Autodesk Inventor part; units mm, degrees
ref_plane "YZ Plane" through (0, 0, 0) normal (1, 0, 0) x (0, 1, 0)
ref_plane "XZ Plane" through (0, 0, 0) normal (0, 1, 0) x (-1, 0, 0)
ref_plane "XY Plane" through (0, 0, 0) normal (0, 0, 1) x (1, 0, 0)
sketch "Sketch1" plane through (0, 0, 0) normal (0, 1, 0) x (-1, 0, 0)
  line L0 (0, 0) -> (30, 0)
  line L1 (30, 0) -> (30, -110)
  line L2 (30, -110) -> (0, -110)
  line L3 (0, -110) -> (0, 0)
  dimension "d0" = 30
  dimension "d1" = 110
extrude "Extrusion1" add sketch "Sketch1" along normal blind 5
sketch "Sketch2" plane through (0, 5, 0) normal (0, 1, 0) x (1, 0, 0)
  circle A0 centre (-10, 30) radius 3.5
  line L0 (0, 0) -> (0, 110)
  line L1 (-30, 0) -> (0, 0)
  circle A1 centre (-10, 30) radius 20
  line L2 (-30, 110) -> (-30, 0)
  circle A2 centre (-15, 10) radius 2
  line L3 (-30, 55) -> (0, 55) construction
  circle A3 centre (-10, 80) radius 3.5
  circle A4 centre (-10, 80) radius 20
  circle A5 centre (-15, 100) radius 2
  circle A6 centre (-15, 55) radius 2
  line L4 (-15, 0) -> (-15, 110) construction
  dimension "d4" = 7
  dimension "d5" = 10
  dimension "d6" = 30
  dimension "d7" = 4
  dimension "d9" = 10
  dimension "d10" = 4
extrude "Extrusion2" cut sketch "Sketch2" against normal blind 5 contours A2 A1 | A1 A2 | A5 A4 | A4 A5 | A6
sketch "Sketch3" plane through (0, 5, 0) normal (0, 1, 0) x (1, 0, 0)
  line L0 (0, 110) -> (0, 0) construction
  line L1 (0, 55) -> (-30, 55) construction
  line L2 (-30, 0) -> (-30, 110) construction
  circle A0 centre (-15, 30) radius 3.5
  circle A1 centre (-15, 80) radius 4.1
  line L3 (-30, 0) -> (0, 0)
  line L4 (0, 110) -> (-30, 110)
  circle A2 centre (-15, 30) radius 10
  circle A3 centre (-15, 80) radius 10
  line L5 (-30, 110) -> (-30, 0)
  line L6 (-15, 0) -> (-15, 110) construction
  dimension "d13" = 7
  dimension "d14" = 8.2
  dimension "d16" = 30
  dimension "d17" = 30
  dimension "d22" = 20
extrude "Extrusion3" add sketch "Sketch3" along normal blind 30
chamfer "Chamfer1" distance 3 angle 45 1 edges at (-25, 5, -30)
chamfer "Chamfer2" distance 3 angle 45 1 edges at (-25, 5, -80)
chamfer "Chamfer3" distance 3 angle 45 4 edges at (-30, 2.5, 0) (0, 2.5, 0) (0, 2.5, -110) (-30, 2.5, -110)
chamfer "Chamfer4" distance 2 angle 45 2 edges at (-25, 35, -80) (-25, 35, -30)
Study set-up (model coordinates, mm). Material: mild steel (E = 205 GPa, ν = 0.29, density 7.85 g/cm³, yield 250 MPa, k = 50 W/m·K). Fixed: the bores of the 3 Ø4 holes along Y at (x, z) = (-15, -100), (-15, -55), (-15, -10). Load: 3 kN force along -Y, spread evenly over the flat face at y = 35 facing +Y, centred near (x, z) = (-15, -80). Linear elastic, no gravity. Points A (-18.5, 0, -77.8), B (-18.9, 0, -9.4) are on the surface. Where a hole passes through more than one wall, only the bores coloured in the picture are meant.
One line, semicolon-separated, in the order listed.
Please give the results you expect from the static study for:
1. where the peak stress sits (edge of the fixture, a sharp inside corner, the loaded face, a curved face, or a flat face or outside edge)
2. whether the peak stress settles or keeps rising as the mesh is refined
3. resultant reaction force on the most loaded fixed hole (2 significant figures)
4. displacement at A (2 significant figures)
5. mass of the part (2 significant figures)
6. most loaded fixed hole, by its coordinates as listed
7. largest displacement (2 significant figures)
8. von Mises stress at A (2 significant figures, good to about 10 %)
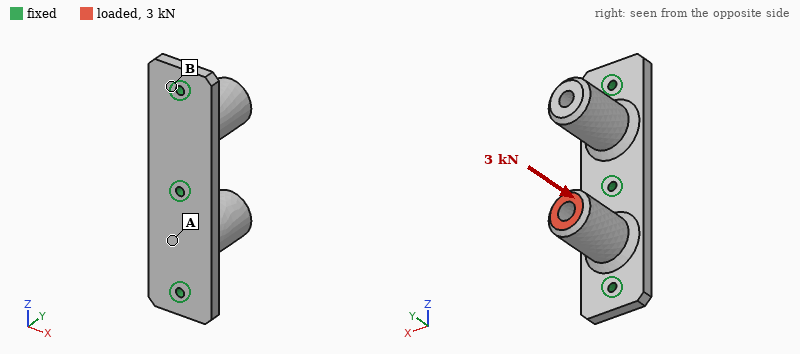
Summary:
edge of the fixture; keeps rising; 1.8 kN; 12 µm; 260 g; (-15, -100); 15 µm; 26 MPa
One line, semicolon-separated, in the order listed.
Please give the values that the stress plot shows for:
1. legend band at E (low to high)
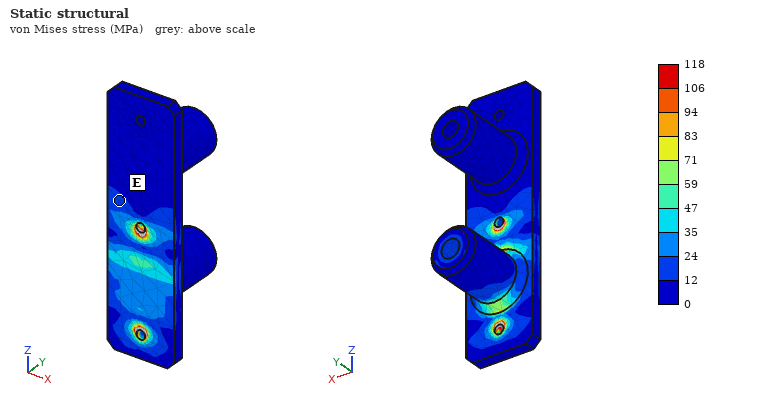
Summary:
12 to 24 MPa
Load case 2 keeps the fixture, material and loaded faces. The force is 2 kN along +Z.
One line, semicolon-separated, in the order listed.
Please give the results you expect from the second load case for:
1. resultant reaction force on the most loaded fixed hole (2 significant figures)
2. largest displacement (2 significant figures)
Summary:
2.1 kN; 43 µm
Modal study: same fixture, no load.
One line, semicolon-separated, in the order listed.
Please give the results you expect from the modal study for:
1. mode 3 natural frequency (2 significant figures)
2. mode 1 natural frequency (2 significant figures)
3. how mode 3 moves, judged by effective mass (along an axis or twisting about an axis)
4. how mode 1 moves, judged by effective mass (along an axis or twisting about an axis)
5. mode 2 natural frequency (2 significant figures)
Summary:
6800 Hz; 3300 Hz; along Z; along X; 3600 Hz
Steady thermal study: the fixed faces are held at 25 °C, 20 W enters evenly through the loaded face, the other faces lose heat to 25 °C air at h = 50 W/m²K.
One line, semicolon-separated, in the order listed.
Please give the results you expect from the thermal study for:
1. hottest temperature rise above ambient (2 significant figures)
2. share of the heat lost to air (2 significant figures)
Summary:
59 K; 35 %
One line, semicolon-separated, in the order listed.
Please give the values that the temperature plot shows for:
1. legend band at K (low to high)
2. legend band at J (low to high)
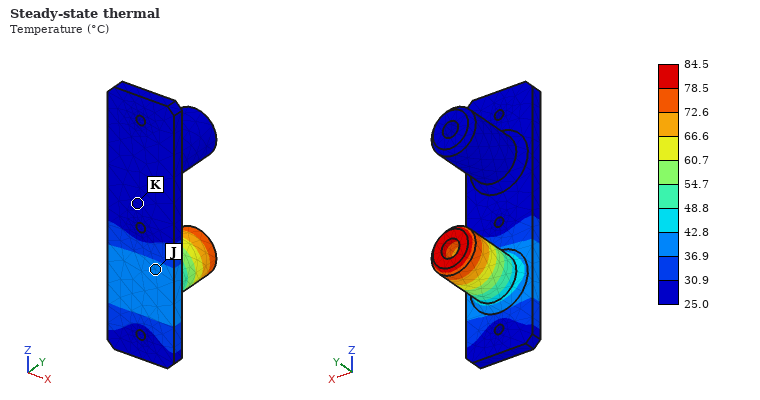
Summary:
25.0 to 30.9 °C; 36.9 to 42.8 °C
